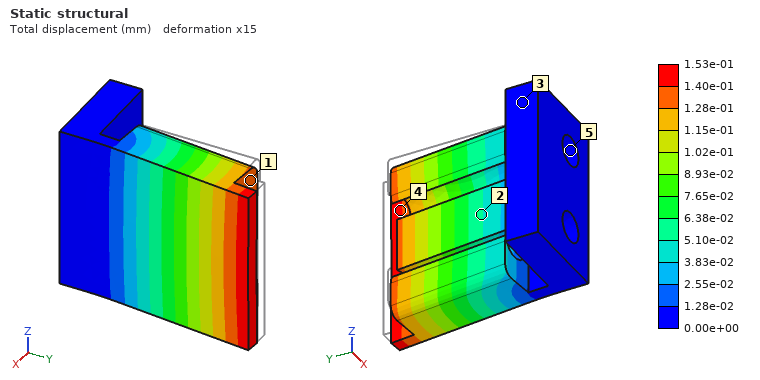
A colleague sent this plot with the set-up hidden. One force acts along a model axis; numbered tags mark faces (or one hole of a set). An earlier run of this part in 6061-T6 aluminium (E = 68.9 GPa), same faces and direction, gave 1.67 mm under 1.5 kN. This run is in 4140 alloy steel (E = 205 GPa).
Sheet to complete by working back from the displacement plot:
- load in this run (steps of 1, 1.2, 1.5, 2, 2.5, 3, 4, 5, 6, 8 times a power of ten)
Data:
400 N
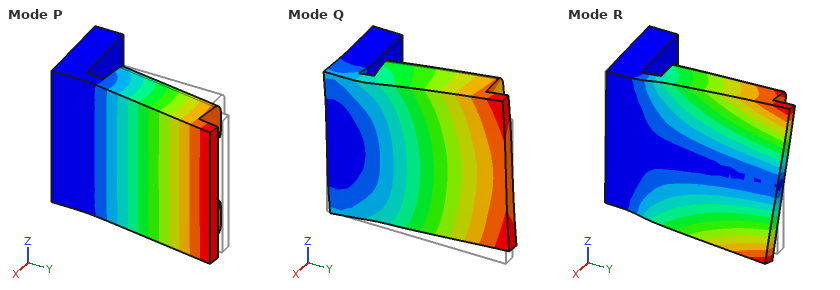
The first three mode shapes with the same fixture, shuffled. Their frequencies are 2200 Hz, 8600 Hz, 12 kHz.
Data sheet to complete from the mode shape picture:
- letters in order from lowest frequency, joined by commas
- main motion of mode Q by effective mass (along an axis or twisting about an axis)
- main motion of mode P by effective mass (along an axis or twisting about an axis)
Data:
P, R, Q
along Z
along X
